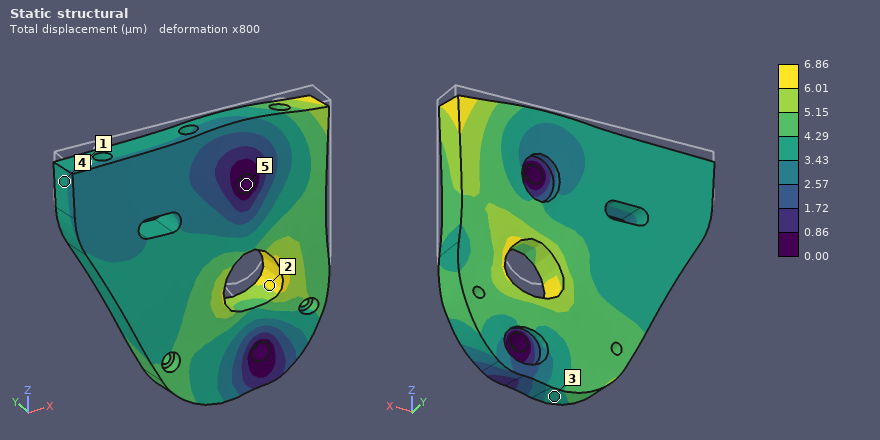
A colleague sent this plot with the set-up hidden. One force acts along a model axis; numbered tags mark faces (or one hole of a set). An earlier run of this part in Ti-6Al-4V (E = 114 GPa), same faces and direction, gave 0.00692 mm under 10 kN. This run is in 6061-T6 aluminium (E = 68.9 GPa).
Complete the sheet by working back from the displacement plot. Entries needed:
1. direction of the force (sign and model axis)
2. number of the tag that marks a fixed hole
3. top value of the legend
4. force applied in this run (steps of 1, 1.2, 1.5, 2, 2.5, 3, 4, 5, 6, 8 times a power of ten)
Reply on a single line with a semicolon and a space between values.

-Z; 5; 6.86 µm; 6 kN
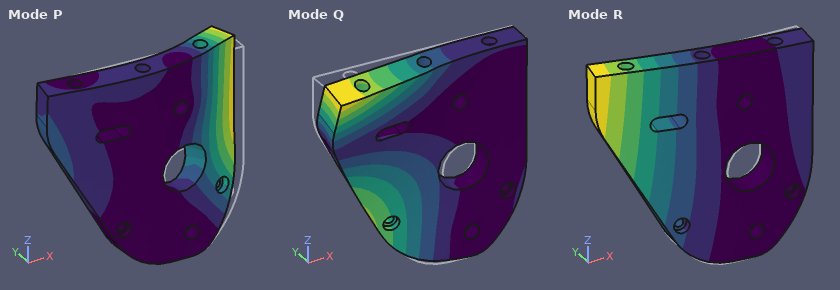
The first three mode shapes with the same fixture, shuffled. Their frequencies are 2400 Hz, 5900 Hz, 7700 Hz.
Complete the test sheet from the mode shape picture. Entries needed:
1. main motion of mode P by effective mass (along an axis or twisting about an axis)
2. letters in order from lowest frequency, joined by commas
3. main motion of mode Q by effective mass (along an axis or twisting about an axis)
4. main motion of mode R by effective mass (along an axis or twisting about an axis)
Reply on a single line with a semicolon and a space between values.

along Y; R, Q, P; twisting about X; along Y
